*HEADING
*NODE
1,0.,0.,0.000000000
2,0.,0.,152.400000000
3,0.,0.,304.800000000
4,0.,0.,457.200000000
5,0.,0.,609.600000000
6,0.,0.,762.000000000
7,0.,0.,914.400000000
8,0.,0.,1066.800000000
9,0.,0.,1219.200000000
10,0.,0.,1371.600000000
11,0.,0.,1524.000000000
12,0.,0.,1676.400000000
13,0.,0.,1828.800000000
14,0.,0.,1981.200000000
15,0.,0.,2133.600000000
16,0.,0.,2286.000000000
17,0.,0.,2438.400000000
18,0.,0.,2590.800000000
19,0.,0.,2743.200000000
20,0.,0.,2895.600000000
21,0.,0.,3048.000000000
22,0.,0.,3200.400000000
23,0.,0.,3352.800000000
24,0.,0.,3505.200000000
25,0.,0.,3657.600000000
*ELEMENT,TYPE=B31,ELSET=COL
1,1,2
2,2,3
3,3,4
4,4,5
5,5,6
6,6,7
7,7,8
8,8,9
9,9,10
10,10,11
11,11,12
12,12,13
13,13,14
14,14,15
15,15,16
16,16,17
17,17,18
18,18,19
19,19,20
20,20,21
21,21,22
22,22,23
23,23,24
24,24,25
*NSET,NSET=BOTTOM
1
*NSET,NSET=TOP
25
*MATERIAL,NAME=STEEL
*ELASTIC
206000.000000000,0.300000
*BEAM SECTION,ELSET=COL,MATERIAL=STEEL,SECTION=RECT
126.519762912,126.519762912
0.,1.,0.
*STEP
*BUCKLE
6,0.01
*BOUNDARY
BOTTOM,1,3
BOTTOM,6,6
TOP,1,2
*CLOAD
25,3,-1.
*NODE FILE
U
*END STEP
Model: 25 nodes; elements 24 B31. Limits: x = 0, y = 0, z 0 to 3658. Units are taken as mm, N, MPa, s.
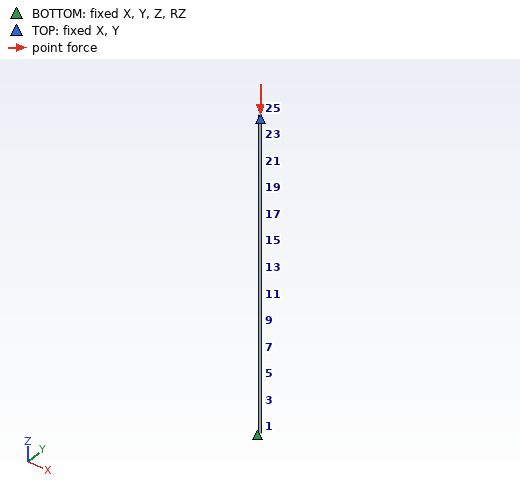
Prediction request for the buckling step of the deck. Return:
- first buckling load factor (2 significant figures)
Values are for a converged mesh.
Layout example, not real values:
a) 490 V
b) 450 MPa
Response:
a) 3.2e+06
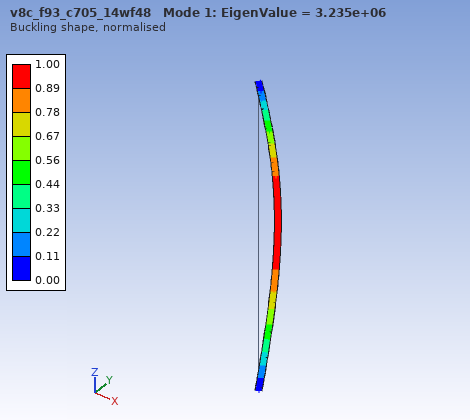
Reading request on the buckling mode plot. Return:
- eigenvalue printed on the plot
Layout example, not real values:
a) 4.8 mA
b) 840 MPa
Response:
a) 3.235e+06
